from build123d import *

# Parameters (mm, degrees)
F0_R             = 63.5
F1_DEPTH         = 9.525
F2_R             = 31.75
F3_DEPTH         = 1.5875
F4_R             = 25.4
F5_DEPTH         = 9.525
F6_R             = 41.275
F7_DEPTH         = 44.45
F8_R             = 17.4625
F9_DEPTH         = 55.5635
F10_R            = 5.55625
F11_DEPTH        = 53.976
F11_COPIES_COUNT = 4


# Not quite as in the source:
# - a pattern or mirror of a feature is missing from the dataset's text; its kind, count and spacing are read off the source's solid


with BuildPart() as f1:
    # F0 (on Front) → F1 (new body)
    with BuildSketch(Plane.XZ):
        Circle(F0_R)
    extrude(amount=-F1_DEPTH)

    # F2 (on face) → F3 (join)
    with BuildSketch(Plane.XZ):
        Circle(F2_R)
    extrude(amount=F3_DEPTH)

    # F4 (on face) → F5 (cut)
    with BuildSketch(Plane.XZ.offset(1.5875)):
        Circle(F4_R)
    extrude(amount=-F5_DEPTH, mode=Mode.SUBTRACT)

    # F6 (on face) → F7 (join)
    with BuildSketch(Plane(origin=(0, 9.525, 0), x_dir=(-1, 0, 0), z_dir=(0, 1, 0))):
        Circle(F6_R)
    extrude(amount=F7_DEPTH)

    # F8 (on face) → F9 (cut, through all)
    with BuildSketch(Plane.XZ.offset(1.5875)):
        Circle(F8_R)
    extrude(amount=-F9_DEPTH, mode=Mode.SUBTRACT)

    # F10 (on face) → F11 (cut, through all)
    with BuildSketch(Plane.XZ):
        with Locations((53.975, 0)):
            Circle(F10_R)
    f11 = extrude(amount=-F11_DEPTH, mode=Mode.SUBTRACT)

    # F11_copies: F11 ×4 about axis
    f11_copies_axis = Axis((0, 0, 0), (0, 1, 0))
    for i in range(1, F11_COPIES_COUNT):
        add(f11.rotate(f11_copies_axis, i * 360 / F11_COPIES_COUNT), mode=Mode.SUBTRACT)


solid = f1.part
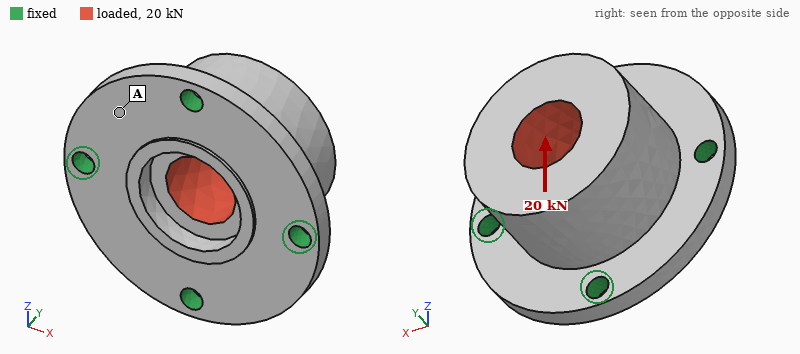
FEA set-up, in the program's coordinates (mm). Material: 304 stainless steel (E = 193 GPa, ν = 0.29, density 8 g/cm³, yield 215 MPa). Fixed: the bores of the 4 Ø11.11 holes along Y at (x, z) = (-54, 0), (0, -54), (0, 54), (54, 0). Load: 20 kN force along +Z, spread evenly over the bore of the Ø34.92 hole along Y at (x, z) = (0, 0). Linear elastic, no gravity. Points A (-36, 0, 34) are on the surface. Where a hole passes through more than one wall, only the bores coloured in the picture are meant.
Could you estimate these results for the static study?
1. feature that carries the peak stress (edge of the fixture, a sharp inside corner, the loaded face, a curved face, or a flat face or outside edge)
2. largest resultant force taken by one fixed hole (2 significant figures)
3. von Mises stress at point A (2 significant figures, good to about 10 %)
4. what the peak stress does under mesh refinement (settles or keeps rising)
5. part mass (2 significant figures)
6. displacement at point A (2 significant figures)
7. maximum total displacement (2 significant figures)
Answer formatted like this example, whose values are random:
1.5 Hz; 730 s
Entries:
edge of the fixture; 8.4 kN; 10.0 MPa; keeps rising; 2.4 kg; 4.9 µm; 13 µm
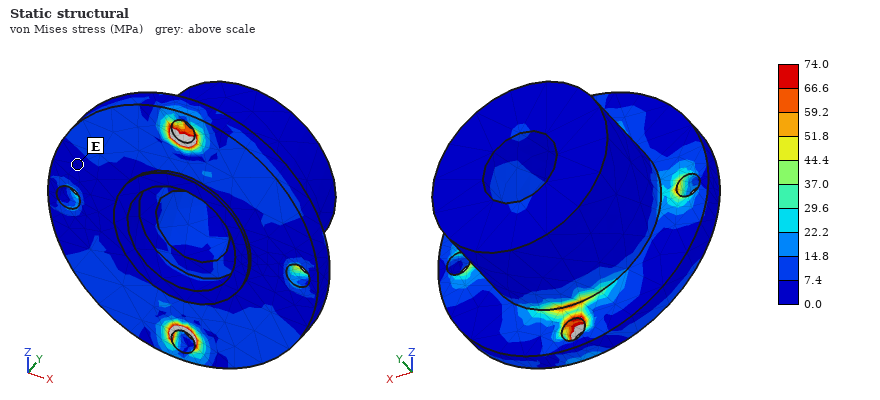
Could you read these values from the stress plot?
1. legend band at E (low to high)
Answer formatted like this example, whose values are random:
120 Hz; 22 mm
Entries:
0.0 to 7.4 MPa
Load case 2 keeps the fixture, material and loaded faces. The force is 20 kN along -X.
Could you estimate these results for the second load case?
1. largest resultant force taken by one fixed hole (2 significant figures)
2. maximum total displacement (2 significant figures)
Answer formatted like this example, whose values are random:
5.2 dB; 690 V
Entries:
8.4 kN; 13 µm
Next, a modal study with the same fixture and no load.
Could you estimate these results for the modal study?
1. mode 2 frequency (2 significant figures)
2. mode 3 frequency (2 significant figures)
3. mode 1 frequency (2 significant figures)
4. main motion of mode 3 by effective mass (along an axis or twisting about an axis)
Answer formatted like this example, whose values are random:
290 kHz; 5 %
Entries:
5200 Hz; 5800 Hz; 5200 Hz; along Y
